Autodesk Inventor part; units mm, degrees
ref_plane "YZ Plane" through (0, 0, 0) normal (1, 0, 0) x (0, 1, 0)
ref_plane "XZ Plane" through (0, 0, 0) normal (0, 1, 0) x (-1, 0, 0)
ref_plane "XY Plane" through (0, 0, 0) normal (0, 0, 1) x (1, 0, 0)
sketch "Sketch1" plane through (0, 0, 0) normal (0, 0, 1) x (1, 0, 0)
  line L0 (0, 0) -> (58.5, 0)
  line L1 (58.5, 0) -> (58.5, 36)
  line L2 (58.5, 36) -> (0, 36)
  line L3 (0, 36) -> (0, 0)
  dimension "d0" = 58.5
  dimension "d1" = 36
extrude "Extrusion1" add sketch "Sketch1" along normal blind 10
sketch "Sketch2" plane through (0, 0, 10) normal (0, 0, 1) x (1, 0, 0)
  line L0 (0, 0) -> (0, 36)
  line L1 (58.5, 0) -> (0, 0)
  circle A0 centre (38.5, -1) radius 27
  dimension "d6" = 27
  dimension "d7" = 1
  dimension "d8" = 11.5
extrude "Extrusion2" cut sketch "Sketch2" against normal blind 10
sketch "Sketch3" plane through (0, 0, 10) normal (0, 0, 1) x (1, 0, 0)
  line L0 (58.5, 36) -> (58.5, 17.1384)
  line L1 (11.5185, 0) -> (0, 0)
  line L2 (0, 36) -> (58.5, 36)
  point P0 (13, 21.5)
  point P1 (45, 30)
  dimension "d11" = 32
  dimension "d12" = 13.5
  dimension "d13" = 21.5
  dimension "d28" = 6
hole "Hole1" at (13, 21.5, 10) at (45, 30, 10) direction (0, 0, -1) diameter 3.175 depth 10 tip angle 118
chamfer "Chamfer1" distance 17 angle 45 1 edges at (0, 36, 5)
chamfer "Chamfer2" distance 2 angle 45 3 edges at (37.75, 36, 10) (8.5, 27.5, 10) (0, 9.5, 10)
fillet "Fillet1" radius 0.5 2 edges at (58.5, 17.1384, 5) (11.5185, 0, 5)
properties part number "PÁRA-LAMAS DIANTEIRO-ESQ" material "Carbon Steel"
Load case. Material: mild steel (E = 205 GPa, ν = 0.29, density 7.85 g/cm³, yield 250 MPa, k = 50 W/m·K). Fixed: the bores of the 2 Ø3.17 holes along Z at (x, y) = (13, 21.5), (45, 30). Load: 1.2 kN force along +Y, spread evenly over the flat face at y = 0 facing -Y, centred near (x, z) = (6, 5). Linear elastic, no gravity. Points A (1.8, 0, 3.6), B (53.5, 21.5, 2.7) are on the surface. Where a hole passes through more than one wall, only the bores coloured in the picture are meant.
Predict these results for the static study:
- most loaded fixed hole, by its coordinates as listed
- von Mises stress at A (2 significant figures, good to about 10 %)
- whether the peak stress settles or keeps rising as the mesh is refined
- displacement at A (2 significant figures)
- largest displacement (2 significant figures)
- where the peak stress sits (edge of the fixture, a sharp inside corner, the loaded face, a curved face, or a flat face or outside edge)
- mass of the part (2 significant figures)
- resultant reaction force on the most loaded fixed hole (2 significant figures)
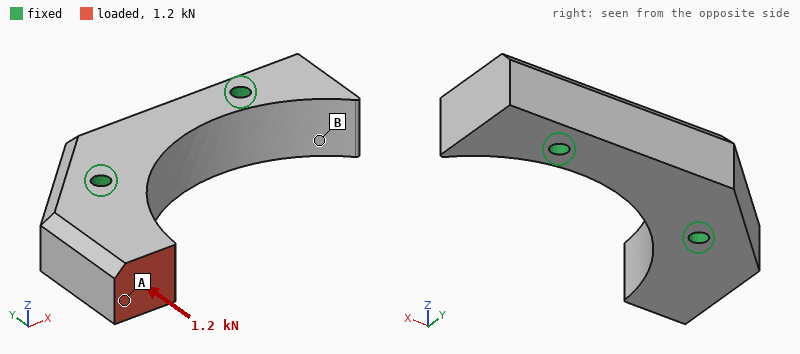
(13, 21.5)
11 MPa
keeps rising
6.8 µm
7.1 µm
edge of the fixture
72 g
1.3 kN
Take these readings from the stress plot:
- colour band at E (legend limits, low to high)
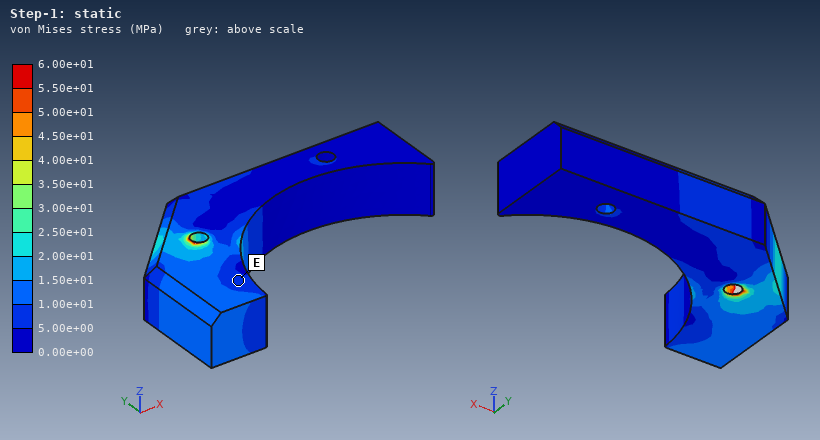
5.00e+00 to 1.00e+01 MPa
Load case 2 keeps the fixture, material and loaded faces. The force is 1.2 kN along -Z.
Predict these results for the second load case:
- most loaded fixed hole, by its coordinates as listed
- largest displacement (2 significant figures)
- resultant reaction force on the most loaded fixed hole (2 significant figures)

(13, 21.5)
29 µm
1.3 kN
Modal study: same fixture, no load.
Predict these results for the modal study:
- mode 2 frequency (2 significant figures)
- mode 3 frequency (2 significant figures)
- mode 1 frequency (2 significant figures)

14 kHz
21 kHz
14 kHz
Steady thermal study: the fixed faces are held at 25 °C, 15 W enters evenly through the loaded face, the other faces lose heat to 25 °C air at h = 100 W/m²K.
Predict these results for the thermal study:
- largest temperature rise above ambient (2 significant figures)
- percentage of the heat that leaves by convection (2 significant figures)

49 K
17 %
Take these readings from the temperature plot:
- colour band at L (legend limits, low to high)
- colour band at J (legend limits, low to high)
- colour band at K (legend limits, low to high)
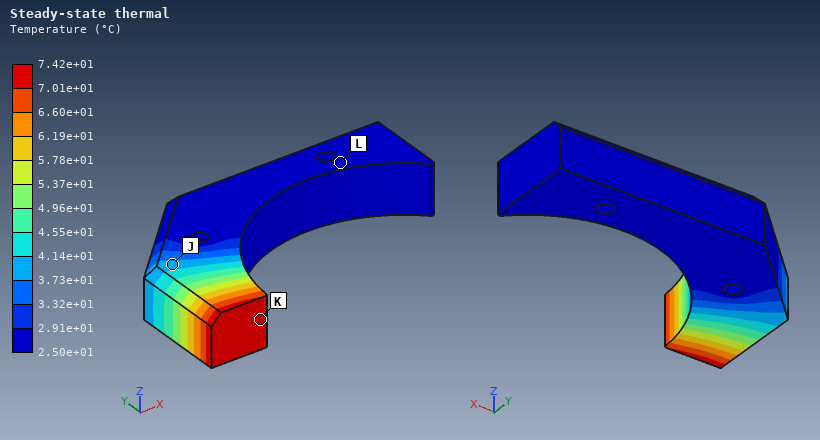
2.50e+01 to 2.91e+01 °C
3.73e+01 to 4.14e+01 °C
7.01e+01 to 7.42e+01 °C
